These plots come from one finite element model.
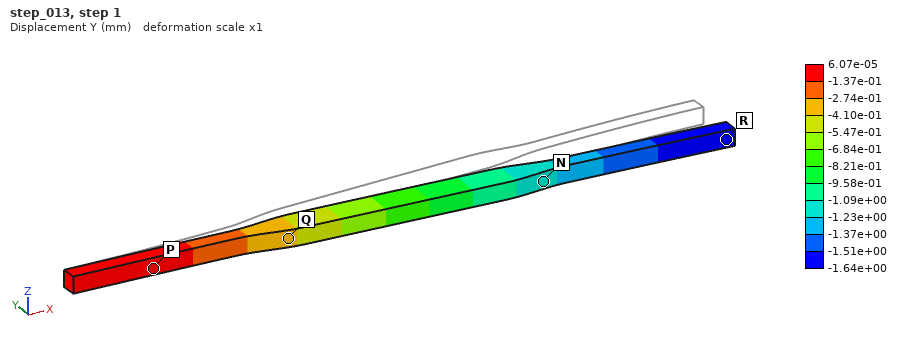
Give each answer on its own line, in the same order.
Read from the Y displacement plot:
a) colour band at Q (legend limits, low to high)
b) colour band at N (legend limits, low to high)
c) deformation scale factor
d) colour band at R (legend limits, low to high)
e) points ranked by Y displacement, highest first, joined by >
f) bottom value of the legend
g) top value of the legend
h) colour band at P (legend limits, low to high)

-4.10e-01 to -2.74e-01 mm
-1.23e+00 to -1.09e+00 mm
1
-1.64e+00 to -1.51e+00 mm
P > Q > N > R
-1.64e+00 mm
6.07e-05 mm
-1.37e-01 to 6.07e-05 mm
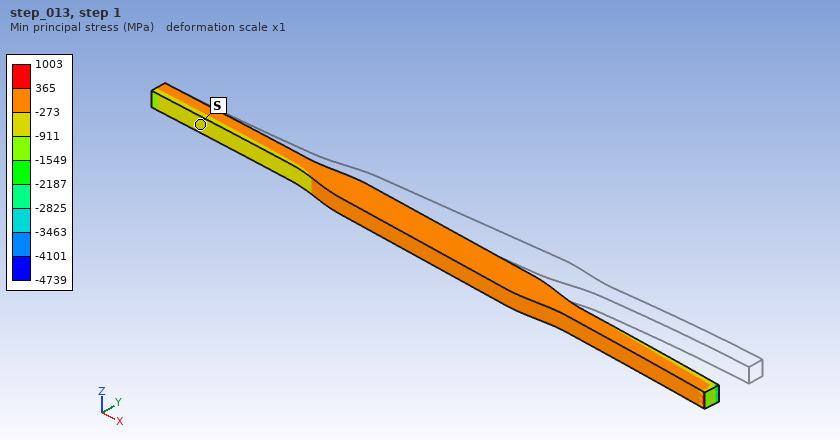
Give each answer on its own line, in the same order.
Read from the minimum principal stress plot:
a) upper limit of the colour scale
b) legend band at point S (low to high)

1003 MPa
-911 to -273 MPa
